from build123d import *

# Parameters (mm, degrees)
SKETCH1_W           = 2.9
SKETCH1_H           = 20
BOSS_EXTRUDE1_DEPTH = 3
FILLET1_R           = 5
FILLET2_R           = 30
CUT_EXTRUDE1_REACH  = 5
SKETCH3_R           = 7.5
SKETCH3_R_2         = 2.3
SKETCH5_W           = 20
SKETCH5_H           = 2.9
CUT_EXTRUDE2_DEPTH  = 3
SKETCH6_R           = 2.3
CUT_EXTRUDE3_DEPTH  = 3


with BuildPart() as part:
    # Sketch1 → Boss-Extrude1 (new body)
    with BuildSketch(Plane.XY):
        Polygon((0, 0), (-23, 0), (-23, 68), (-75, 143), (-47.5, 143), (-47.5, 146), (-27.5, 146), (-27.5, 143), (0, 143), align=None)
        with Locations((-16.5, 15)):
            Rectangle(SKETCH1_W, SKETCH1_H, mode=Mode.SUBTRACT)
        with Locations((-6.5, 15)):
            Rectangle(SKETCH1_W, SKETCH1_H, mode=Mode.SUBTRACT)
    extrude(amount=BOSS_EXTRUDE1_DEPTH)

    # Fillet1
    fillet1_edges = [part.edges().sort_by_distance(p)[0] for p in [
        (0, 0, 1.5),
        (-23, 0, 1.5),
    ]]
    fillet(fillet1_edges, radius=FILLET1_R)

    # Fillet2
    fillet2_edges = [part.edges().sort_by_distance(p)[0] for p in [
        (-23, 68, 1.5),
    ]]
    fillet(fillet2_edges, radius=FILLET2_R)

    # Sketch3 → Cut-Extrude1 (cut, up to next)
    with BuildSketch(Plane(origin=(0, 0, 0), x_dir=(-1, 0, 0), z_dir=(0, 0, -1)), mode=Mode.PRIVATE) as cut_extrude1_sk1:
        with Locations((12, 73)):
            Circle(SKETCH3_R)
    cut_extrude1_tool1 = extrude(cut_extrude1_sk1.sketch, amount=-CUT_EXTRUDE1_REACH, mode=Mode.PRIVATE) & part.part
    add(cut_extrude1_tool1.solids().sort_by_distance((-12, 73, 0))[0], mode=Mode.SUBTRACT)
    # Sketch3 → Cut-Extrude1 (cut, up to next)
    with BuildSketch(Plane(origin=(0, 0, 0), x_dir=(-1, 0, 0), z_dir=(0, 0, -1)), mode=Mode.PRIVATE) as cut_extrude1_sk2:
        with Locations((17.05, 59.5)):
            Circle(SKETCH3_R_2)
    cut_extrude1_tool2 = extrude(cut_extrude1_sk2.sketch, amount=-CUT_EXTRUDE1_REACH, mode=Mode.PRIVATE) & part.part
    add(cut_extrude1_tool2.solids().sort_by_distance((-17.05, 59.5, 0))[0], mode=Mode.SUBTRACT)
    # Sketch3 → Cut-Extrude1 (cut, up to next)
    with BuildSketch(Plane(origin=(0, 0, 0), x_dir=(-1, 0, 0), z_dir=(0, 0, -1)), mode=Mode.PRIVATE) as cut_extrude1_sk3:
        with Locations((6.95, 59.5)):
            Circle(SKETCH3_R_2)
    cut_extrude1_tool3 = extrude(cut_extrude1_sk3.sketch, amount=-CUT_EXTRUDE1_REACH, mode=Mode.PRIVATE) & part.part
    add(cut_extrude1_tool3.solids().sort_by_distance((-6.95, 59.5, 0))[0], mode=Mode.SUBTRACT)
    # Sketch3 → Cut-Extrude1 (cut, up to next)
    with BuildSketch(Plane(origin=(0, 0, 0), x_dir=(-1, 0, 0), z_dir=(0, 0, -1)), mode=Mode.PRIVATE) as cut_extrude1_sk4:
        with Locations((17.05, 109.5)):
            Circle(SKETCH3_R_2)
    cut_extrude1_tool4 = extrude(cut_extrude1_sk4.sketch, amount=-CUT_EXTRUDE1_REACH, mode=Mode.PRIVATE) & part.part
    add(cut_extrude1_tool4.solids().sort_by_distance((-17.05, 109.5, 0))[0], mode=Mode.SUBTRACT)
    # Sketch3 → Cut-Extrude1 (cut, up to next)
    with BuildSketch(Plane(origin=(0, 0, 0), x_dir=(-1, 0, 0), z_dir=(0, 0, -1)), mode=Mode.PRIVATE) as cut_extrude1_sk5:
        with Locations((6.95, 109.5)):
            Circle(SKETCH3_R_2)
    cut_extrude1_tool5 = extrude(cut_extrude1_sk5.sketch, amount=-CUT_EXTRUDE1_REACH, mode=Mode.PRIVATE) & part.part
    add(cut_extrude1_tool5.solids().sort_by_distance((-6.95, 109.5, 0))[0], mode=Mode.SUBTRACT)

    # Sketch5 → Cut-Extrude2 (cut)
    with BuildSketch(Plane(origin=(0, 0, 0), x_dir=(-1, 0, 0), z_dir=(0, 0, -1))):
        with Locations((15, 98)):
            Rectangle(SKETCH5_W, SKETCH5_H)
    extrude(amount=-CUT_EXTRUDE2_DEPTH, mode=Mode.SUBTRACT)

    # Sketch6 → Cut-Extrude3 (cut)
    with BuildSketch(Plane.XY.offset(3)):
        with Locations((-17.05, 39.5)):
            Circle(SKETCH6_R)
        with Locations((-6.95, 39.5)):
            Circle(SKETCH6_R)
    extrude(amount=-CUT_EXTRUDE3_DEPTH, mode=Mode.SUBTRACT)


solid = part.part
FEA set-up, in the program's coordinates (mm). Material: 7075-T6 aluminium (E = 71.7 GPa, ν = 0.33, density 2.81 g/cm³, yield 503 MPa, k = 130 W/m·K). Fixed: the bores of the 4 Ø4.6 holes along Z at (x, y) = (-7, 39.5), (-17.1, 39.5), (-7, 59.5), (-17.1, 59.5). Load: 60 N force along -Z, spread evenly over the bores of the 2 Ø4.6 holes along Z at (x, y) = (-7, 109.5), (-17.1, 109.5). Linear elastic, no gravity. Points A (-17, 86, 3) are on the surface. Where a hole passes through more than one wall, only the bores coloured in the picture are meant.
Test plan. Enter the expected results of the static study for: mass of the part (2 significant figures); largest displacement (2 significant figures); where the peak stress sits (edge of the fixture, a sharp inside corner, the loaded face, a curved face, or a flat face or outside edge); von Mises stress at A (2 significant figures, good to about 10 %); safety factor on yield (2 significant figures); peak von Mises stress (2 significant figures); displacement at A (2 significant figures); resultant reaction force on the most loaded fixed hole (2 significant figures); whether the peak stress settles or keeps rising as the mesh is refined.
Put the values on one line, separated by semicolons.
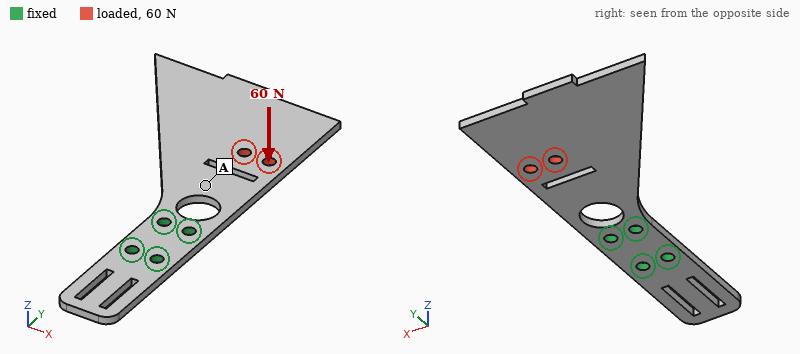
41 g; 1.9 mm; a curved face; 22 MPa; 2.9; 170 MPa; 0.34 mm; 32 N; settles
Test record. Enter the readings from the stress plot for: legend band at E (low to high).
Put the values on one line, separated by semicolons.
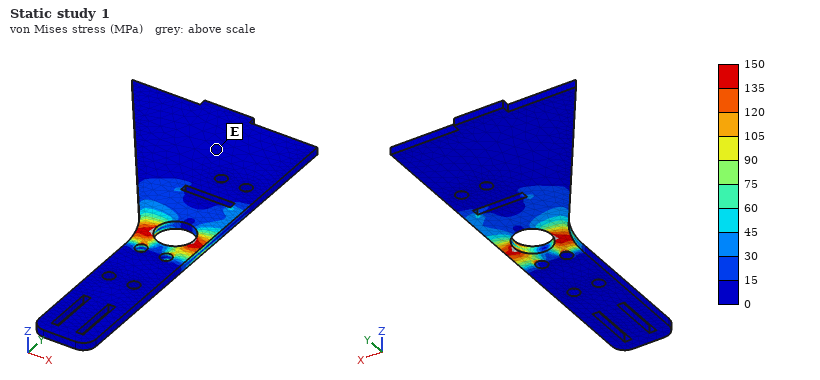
0 to 15 MPa
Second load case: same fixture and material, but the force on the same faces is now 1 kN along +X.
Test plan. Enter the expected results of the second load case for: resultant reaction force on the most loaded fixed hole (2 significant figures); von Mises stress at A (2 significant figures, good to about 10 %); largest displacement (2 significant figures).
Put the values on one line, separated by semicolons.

2.6 kN; 57 MPa; 0.68 mm
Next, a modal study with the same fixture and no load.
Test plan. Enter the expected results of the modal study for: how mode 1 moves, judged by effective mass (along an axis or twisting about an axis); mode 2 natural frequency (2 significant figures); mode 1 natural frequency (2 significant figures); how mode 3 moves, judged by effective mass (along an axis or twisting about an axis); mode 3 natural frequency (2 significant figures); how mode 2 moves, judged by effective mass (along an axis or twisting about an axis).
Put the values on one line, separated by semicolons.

along Z; 640 Hz; 170 Hz; along X; 1300 Hz; twisting about Y
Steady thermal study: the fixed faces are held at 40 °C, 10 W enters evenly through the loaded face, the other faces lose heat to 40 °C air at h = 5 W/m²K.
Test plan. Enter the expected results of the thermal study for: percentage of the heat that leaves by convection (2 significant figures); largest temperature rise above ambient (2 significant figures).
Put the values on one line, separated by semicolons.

19 %; 61 K
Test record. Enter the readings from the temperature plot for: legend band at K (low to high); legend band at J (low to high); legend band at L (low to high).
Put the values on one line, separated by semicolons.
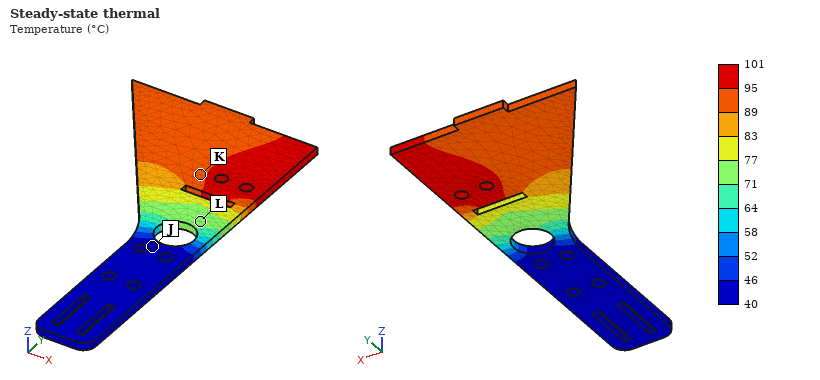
89 to 95 °C; 40 to 46 °C; 71 to 77 °C
